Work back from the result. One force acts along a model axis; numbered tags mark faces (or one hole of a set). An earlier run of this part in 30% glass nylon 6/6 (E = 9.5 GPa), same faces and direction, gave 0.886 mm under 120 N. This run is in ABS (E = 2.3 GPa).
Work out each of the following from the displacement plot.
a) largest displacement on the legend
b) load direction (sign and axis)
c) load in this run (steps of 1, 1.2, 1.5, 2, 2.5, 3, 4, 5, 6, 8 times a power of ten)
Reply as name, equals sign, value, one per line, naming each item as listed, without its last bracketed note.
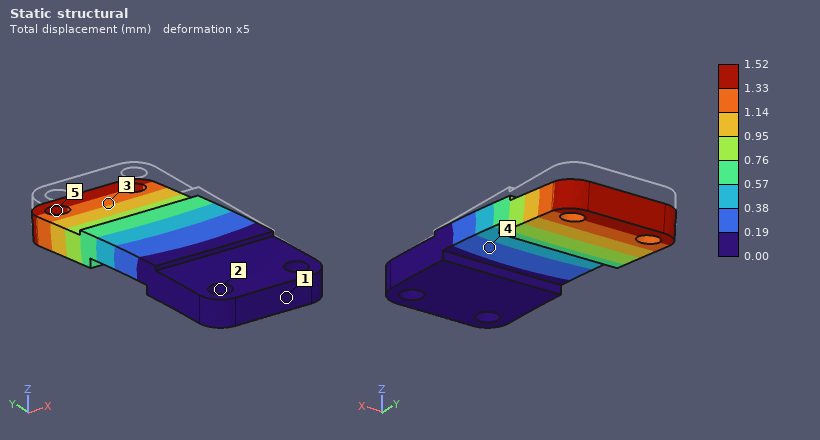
largest displacement on the legend = 1.52 mm
load direction = -Z
load in this run = 50 N
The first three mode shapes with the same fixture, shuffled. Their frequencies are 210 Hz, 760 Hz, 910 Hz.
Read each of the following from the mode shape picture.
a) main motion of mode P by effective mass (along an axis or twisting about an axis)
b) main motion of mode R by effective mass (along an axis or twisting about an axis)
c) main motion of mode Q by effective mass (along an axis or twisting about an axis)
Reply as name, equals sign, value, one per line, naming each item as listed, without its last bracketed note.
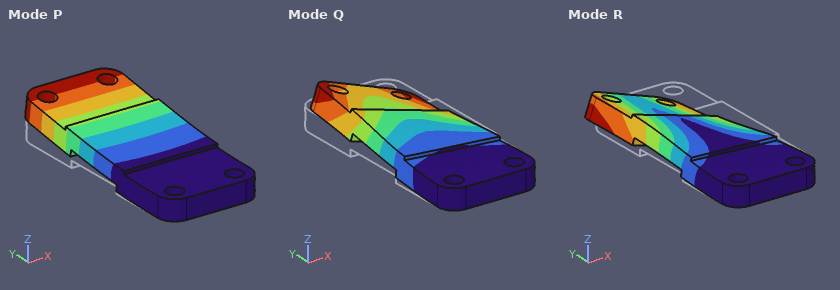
main motion of mode P by effective mass = along Z
main motion of mode R by effective mass = along X
main motion of mode Q by effective mass = along X
